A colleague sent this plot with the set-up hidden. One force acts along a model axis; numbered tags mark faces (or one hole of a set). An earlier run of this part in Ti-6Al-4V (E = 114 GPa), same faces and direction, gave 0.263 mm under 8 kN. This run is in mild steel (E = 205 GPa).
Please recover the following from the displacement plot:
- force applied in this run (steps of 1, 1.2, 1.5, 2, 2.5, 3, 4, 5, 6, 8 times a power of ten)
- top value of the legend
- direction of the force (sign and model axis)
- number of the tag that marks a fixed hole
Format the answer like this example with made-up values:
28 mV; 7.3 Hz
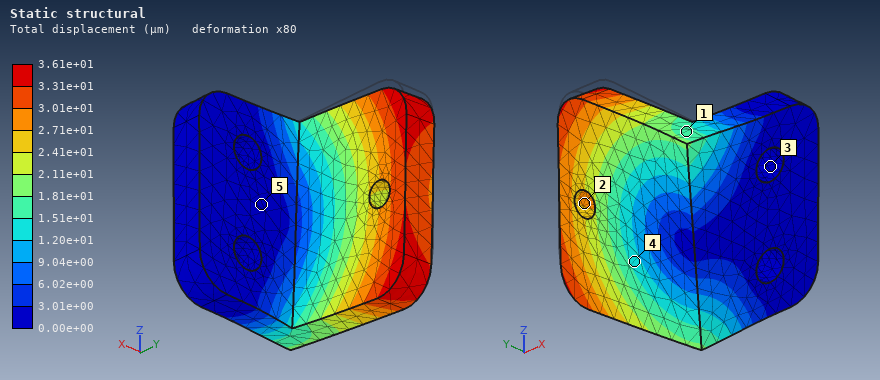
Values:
2 kN; 3.61e+01 µm; -Z; 3
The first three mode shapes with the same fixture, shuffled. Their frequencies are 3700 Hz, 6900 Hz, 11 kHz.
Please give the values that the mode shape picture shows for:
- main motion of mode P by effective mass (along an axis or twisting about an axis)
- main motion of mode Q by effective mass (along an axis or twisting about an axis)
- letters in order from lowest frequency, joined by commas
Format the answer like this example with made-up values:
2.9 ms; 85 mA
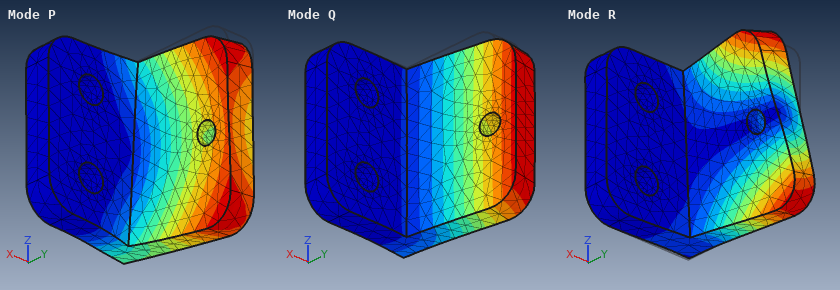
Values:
along Z; along X; Q, P, R
